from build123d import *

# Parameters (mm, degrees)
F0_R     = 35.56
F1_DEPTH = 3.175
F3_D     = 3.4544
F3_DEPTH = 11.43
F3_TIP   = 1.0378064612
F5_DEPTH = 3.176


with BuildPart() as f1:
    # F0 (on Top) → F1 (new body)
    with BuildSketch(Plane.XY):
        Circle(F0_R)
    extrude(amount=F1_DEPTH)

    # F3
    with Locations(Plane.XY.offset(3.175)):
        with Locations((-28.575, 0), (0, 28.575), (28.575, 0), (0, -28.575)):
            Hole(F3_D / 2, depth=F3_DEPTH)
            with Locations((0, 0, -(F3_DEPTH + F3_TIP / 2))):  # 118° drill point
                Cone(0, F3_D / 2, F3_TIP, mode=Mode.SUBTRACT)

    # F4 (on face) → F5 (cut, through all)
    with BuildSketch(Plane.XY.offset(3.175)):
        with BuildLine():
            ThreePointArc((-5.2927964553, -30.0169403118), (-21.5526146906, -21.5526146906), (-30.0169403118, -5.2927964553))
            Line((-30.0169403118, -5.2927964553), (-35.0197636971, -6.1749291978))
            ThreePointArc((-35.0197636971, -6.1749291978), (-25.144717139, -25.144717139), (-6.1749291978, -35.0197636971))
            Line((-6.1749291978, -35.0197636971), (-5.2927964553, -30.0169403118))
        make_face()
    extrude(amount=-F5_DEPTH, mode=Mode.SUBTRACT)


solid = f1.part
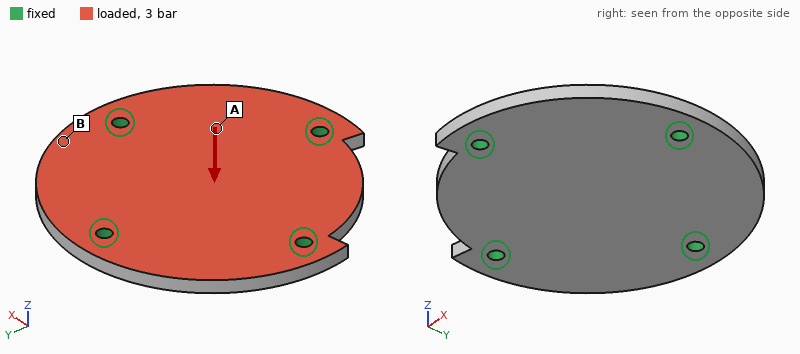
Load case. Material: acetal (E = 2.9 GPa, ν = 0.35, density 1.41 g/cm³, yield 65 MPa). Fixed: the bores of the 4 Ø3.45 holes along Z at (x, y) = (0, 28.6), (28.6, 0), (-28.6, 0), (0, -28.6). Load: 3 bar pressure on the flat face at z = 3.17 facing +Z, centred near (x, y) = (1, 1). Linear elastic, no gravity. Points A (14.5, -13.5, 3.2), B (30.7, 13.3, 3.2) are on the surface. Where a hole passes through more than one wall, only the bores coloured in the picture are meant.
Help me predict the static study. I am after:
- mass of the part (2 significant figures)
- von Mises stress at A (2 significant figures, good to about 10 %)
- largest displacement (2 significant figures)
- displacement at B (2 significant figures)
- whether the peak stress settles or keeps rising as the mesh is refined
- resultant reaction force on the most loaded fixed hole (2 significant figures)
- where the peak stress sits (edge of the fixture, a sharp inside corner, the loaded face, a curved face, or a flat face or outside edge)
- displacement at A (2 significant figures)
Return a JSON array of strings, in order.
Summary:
["17 g", "15 MPa", "0.57 mm", "0.24 mm", "keeps rising", "300 N", "edge of the fixture", "0.40 mm"]
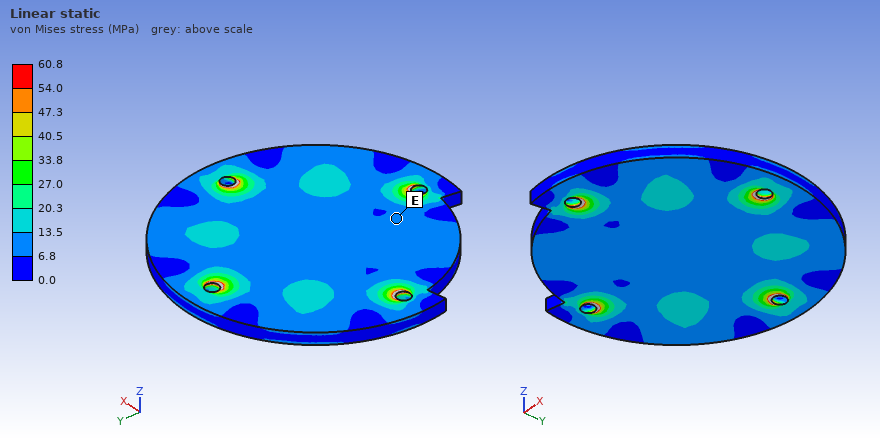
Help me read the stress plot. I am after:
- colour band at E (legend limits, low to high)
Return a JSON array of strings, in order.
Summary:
["6.8 to 13.5 MPa"]
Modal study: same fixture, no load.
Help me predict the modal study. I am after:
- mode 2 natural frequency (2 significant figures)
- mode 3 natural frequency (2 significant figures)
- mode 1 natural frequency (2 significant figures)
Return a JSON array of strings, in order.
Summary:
["2100 Hz", "2200 Hz", "2000 Hz"]
